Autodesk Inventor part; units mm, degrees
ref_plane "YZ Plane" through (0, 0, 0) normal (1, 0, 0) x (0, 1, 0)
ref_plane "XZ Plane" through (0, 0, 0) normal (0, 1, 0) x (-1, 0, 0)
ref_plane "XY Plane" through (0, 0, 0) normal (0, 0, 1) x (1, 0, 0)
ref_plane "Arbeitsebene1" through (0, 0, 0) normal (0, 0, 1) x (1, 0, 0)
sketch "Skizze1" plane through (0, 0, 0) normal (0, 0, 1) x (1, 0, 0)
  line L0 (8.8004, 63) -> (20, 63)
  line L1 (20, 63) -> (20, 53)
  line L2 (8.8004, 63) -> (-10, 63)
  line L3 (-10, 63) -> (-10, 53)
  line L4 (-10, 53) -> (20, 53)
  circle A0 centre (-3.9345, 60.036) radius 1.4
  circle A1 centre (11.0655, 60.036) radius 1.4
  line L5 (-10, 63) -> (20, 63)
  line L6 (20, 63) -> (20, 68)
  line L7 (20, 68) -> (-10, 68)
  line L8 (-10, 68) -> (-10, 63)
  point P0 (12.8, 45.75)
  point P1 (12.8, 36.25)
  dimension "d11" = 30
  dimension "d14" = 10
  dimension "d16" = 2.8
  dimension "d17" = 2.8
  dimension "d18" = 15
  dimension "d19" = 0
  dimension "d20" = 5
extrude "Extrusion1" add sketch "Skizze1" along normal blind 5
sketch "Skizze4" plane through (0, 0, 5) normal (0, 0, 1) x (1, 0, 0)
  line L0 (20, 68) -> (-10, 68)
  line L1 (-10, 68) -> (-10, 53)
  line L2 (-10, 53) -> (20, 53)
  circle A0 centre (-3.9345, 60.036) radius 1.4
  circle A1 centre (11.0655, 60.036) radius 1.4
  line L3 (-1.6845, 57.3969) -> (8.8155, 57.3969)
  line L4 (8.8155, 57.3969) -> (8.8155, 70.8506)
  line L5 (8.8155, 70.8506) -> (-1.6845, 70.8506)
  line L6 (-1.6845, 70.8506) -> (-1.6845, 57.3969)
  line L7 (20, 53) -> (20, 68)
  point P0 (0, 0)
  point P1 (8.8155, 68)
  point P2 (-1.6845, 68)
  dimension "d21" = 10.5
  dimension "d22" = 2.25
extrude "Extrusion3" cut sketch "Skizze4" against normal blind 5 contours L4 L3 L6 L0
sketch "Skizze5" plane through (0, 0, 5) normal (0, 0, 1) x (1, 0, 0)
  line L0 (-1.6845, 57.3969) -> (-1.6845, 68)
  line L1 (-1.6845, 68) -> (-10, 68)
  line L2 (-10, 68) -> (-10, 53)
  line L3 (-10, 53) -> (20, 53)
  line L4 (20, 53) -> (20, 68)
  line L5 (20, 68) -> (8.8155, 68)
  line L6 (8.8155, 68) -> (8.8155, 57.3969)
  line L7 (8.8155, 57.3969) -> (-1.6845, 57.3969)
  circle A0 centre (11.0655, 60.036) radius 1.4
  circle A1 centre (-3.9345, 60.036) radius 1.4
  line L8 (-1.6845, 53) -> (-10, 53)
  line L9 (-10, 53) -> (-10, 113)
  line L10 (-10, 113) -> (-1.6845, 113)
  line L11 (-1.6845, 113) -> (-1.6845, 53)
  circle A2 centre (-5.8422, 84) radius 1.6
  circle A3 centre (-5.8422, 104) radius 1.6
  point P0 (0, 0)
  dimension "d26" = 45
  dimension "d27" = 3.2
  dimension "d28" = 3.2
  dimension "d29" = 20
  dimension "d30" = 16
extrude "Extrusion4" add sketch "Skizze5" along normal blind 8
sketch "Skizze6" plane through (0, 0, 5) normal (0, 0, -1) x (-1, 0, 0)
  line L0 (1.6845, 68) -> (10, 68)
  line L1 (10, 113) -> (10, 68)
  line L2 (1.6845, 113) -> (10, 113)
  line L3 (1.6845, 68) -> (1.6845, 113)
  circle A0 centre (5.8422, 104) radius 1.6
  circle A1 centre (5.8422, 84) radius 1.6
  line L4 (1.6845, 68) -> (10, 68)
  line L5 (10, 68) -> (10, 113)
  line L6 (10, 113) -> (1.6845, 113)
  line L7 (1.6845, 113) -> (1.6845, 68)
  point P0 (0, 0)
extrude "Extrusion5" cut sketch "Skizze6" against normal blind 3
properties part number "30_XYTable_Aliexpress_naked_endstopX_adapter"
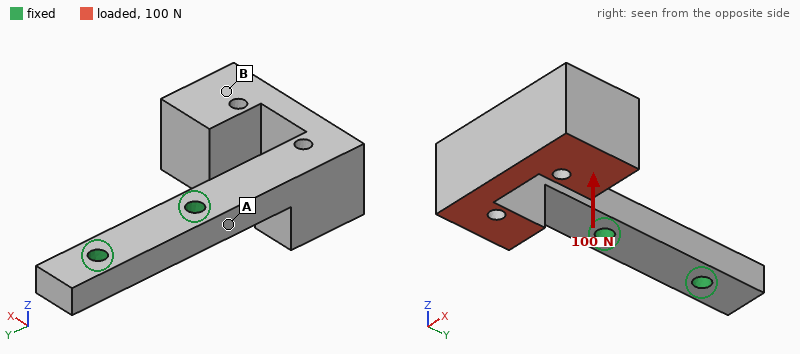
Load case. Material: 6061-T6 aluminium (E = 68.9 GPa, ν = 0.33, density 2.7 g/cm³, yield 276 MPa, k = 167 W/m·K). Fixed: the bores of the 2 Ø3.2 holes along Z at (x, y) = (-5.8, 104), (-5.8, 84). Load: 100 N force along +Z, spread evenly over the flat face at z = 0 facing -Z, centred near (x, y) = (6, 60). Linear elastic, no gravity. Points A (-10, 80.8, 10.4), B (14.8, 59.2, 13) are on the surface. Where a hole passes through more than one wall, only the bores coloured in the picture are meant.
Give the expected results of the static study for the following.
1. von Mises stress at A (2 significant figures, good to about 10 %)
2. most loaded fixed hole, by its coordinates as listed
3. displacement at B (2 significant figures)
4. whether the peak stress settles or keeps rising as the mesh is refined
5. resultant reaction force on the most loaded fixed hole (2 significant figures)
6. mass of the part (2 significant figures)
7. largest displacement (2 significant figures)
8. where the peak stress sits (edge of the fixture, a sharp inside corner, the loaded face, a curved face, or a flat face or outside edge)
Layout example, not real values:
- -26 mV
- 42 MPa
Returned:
- 37 MPa
- (-5.8, 84)
- 0.16 mm
- keeps rising
- 110 N
- 16 g
- 0.21 mm
- edge of the fixture
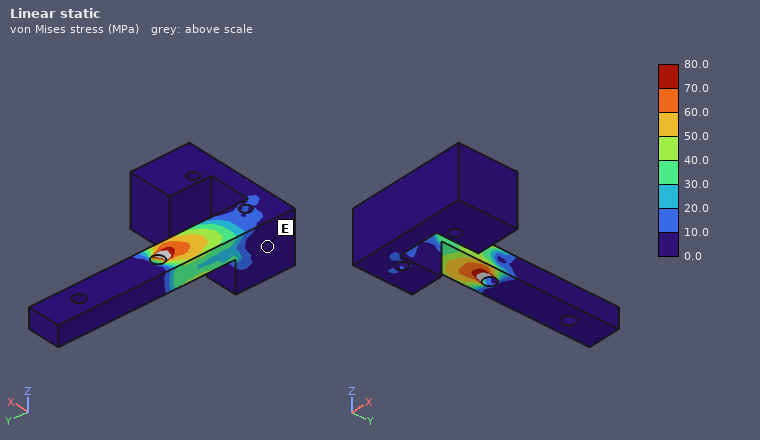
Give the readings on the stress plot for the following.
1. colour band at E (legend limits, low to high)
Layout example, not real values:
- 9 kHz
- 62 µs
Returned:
- 0.0 to 10.0 MPa
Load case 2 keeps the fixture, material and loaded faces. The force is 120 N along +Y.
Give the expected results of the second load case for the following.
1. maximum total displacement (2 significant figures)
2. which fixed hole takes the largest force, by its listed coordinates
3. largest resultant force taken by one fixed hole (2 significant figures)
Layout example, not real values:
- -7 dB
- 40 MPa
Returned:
- 0.16 mm
- (-5.8, 84)
- 120 N
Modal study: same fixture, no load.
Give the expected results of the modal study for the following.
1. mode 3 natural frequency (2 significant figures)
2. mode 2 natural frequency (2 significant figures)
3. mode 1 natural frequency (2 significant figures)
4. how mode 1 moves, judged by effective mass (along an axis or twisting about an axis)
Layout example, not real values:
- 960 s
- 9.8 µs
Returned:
- 2800 Hz
- 1700 Hz
- 1200 Hz
- along Z
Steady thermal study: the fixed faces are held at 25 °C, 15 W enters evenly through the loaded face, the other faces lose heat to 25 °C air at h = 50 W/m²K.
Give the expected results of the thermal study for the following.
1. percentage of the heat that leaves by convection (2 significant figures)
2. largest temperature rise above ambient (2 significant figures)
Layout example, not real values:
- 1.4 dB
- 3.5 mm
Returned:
- 27 %
- 47 K
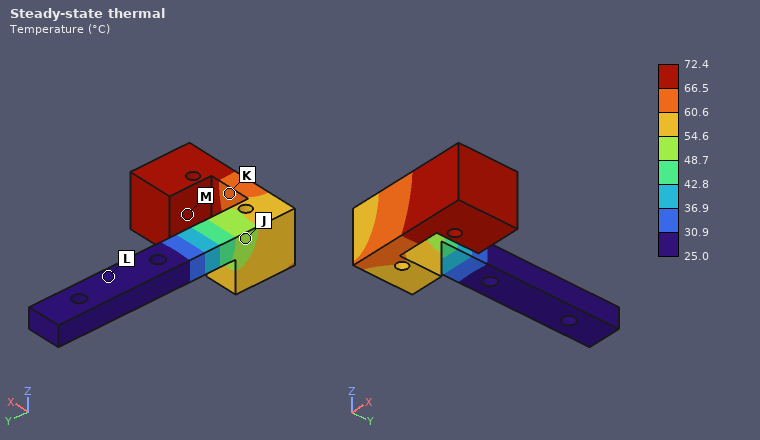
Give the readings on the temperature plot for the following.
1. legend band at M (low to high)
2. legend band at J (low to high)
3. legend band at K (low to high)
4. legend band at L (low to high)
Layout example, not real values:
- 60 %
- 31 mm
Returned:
- 66.5 to 72.4 °C
- 48.7 to 54.6 °C
- 60.6 to 66.5 °C
- 25.0 to 30.9 °C
